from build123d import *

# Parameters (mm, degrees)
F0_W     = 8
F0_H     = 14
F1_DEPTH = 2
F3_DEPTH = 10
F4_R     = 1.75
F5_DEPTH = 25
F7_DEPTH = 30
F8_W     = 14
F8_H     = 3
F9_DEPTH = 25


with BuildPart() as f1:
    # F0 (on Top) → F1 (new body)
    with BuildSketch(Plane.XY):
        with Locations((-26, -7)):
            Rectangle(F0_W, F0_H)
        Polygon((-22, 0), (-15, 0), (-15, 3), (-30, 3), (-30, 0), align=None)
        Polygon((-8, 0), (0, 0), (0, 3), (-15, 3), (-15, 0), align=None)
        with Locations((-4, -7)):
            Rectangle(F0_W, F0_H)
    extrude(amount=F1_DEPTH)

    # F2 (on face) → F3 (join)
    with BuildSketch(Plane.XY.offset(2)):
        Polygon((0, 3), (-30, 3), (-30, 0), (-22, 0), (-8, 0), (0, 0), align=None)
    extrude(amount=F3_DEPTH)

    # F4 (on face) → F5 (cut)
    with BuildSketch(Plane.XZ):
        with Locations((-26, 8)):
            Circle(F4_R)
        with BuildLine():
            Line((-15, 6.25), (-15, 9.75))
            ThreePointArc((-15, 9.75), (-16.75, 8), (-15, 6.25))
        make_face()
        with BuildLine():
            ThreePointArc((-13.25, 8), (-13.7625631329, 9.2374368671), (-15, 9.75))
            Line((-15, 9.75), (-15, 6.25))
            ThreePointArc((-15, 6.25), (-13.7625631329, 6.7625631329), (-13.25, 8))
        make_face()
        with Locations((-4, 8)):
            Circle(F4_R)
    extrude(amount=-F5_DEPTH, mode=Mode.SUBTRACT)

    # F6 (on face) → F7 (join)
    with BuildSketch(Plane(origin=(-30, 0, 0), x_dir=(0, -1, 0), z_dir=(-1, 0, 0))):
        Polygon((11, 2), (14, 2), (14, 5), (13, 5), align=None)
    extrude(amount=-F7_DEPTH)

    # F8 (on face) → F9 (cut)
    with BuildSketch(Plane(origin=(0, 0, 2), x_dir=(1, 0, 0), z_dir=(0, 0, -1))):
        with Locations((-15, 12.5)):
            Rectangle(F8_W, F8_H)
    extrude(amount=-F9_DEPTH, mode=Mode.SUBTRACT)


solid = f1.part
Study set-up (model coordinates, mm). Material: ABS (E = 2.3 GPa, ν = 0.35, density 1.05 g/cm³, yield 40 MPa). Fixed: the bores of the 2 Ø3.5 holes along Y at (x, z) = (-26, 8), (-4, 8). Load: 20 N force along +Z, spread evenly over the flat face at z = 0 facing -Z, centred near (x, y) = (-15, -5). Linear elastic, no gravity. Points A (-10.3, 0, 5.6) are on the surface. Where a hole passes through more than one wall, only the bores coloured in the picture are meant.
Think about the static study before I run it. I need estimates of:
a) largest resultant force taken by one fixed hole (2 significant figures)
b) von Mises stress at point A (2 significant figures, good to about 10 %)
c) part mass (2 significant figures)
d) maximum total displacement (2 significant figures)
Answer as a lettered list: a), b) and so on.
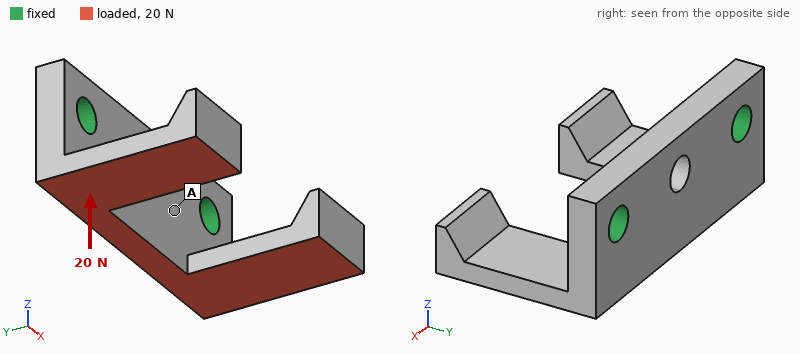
a) 10 N
b) 1.3 MPa
c) 1.6 g
d) 0.35 mm
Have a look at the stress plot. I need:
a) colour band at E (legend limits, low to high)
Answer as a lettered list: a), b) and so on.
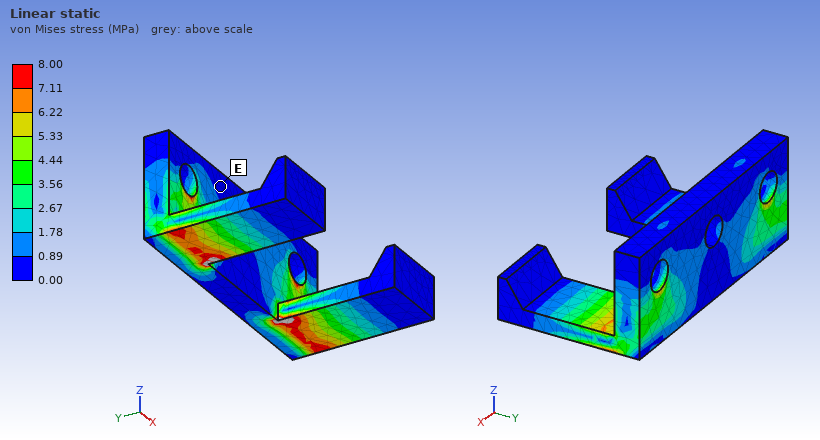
a) 0.00 to 0.89 MPa
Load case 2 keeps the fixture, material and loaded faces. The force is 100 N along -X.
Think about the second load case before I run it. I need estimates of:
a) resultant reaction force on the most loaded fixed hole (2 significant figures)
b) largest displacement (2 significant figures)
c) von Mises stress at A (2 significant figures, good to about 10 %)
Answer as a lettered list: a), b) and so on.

a) 59 N
b) 0.37 mm
c) 2.5 MPa
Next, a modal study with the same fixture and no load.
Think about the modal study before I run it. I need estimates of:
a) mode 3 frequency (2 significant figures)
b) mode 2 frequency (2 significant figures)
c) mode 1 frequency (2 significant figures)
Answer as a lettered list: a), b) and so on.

a) 2700 Hz
b) 1500 Hz
c) 1400 Hz
